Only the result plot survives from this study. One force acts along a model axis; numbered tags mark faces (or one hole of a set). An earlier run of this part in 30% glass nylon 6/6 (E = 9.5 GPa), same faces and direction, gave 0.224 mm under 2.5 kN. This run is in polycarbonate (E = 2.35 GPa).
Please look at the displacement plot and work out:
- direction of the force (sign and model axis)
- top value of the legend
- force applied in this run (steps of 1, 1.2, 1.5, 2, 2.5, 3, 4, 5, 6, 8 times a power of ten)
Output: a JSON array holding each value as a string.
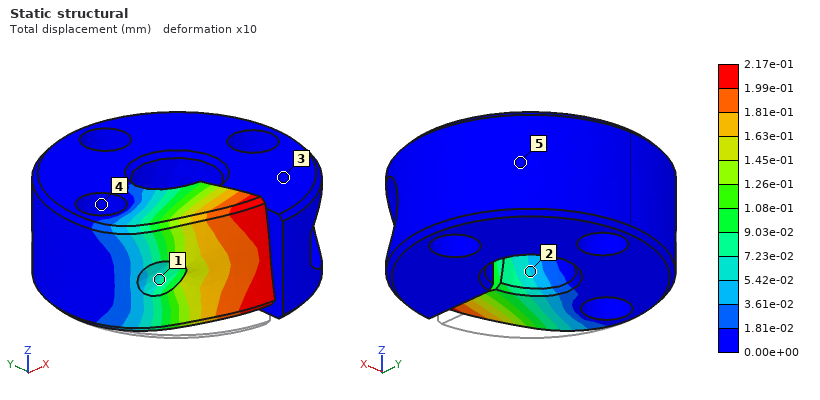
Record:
["+Z", "2.17e-01 mm", "600 N"]
